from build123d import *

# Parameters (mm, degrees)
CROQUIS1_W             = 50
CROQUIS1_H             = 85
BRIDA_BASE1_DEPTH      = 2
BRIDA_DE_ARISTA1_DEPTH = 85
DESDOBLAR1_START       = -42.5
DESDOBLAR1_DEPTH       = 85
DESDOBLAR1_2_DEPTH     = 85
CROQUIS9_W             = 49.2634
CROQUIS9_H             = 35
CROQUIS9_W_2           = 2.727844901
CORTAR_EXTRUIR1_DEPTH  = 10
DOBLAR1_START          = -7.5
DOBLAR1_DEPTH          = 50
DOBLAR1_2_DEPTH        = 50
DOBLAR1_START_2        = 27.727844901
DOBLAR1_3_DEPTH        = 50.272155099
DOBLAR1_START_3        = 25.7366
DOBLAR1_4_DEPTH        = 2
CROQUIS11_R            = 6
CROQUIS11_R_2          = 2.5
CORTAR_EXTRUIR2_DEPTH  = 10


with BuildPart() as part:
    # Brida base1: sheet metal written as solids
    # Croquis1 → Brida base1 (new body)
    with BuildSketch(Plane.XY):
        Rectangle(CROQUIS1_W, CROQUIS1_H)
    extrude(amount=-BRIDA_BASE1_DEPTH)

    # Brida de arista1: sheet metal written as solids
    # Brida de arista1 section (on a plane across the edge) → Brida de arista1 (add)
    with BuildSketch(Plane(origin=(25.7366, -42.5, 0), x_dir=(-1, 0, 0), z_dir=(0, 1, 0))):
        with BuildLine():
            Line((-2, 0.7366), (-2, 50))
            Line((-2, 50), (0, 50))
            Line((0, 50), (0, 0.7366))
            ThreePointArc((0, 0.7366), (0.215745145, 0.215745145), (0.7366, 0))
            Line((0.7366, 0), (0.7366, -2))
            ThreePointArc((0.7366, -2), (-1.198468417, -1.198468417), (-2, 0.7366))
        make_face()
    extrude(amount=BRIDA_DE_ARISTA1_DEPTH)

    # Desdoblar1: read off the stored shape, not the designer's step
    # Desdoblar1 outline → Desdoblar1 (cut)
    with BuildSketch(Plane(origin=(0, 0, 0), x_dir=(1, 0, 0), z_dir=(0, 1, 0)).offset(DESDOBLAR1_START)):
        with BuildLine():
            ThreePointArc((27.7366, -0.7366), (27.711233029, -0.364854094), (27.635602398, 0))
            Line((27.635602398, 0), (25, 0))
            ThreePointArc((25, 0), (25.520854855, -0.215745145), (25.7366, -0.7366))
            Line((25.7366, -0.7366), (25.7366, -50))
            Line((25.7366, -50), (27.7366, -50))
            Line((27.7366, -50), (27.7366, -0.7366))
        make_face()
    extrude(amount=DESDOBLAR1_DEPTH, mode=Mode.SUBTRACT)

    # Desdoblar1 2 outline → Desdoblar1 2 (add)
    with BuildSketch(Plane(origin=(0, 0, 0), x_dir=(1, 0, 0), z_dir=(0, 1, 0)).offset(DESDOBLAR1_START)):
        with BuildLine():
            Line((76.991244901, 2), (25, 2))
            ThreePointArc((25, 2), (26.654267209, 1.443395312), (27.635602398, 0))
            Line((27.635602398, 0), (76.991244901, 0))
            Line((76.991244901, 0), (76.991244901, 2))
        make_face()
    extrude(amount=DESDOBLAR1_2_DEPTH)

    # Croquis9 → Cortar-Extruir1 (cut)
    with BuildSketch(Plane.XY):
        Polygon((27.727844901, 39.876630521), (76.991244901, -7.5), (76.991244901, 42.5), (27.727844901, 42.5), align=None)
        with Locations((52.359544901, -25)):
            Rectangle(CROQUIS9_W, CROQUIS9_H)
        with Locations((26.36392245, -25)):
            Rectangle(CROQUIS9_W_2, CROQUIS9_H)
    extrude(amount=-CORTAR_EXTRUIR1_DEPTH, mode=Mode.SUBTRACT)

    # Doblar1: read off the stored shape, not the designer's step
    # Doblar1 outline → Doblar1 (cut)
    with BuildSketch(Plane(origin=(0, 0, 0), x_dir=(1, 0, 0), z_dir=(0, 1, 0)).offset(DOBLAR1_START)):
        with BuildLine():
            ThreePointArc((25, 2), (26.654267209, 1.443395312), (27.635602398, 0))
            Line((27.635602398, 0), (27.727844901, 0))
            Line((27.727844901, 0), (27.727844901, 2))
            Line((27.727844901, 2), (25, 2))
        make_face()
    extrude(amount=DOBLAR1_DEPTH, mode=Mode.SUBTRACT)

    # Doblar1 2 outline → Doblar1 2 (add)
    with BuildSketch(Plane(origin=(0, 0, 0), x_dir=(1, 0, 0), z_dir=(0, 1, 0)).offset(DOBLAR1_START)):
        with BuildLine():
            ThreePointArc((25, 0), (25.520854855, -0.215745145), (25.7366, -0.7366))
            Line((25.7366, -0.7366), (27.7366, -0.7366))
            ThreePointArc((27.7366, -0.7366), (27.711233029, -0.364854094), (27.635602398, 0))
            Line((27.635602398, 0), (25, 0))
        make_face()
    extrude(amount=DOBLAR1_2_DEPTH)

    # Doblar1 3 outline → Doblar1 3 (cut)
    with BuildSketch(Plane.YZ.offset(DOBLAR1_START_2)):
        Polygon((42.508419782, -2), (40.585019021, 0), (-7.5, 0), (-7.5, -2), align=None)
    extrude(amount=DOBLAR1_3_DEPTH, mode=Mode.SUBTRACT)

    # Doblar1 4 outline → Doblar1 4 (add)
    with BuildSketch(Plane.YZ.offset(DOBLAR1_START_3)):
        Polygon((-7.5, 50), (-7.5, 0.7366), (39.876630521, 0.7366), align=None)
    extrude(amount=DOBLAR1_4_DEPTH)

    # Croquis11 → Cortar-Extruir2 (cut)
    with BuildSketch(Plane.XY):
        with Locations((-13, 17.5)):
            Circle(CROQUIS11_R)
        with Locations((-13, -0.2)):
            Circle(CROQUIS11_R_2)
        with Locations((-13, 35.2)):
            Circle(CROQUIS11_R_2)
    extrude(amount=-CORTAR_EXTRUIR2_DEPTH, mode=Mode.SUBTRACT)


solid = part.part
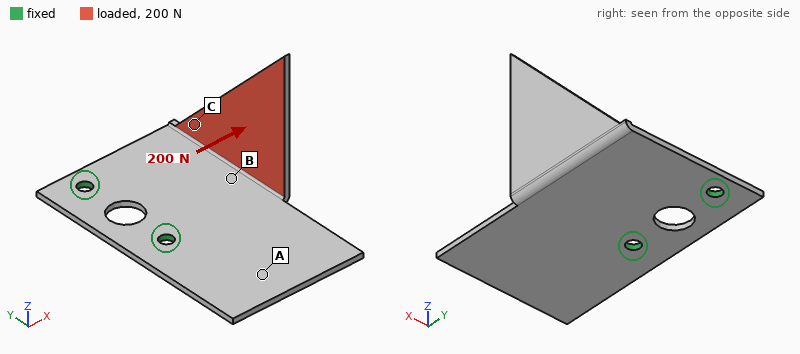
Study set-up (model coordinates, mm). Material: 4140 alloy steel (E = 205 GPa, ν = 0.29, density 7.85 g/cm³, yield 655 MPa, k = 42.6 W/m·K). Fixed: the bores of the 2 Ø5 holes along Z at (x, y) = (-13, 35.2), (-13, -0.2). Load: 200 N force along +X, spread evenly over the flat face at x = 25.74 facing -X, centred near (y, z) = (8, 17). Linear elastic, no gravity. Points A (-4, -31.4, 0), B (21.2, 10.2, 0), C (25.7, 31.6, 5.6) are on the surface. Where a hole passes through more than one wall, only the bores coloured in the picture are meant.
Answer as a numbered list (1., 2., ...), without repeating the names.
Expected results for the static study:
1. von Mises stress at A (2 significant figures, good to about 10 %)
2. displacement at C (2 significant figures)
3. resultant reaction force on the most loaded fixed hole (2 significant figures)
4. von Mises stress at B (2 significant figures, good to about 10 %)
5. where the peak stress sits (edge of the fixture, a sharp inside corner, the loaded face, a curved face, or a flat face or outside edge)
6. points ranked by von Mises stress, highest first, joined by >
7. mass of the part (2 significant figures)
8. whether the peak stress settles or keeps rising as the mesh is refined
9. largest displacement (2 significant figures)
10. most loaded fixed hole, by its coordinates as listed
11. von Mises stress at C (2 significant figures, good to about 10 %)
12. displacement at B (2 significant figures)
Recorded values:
1. 31 MPa
2. 0.31 mm
3. 150 N
4. 100 MPa
5. a sharp inside corner
6. B > C > A
7. 85 g
8. keeps rising
9. 1.3 mm
10. (-13, -0.2)
11. 68 MPa
12. 0.23 mm
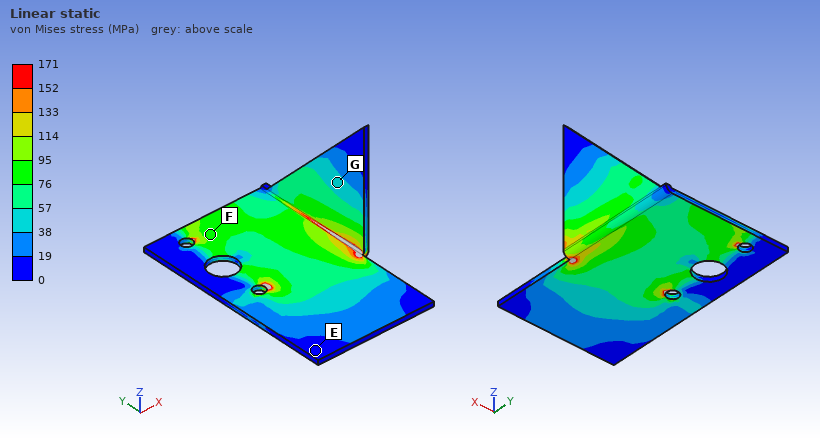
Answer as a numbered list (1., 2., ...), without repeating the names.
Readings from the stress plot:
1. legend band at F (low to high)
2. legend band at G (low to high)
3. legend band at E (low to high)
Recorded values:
1. 76 to 95 MPa
2. 38 to 57 MPa
3. 0 to 19 MPa
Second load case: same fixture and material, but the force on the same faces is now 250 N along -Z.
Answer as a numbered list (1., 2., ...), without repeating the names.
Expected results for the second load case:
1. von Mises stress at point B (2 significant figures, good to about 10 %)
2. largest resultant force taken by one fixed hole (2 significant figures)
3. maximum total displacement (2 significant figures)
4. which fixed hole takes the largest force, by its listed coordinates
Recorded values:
1. 24 MPa
2. 180 N
3. 1.2 mm
4. (-13, -0.2)
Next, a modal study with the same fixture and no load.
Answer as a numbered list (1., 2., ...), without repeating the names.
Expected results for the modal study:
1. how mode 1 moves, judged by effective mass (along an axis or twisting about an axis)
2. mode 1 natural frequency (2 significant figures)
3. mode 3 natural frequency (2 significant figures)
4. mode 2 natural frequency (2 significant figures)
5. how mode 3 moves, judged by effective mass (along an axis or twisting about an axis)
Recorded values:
1. along Z
2. 480 Hz
3. 1100 Hz
4. 750 Hz
5. along Z
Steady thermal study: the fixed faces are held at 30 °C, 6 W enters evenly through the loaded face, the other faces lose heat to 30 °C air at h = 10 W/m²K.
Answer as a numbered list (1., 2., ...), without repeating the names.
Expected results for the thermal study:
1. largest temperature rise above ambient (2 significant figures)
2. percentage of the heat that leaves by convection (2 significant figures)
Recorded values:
1. 75 K
2. 35 %
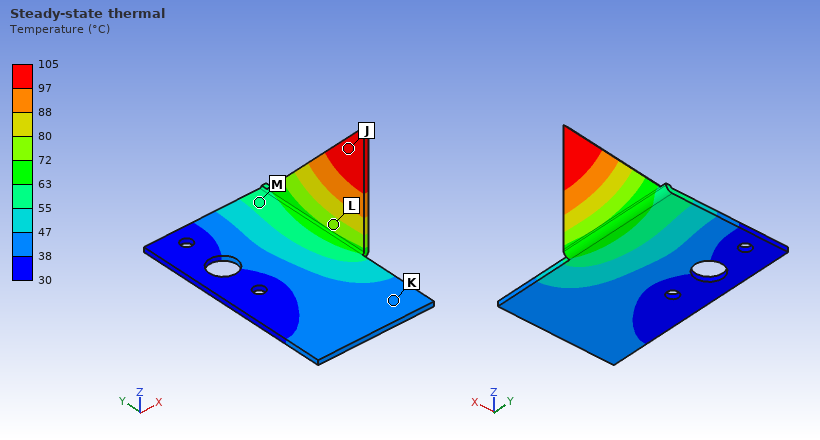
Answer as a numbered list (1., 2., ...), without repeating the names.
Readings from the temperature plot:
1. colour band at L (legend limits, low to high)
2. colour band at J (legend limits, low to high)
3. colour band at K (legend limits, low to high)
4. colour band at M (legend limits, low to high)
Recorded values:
1. 72 to 80 °C
2. 97 to 105 °C
3. 38 to 47 °C
4. 55 to 63 °C
